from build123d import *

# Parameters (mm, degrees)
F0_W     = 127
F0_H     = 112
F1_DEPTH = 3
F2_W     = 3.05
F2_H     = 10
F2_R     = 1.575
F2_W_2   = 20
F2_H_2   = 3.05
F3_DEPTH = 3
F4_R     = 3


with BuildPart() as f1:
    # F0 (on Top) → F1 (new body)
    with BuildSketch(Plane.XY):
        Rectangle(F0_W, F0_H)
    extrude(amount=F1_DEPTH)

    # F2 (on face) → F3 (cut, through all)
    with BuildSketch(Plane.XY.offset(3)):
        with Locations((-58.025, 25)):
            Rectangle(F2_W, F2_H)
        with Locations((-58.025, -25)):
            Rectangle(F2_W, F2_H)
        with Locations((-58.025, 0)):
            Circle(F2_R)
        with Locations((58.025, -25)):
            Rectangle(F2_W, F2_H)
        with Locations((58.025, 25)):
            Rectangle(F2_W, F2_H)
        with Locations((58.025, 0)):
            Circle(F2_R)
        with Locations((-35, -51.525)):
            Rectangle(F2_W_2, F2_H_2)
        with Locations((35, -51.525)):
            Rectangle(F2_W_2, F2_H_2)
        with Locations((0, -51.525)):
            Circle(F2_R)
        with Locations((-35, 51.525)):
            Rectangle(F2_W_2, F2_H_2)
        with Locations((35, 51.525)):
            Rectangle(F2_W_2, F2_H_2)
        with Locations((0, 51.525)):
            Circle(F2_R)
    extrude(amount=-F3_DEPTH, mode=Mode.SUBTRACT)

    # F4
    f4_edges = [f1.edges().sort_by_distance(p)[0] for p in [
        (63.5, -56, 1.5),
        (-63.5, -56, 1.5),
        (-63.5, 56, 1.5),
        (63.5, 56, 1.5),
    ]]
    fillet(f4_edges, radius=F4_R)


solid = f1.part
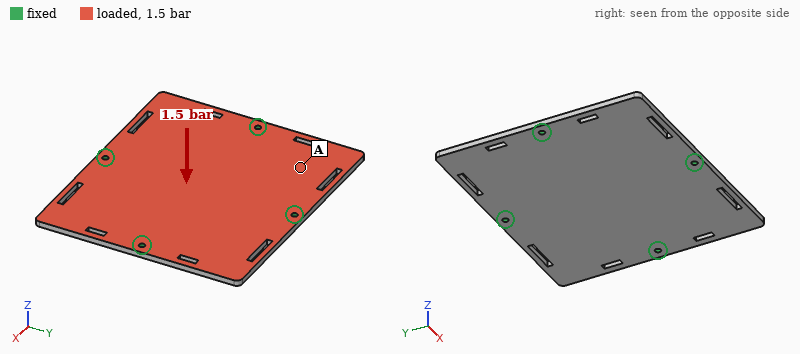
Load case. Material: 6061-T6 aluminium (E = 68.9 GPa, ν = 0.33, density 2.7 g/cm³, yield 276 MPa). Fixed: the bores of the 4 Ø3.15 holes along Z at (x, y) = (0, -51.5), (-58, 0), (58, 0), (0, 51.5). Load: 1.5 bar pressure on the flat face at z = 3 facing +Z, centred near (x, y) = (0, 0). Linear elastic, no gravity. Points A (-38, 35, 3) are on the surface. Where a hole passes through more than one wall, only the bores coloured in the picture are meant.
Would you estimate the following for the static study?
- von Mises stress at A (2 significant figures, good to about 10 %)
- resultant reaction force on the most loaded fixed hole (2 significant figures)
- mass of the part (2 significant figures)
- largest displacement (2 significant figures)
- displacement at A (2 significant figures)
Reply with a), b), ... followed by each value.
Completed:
a) 38 MPa
b) 520 N
c) 110 g
d) 0.38 mm
e) 0.19 mm
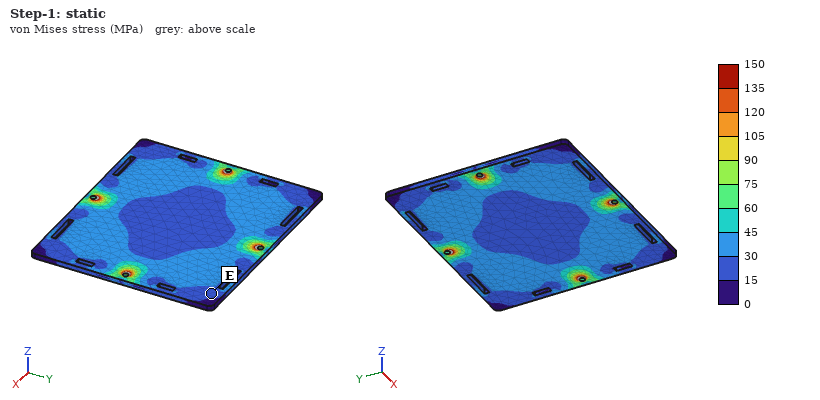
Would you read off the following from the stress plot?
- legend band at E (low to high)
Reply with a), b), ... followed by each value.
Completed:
a) 15 to 30 MPa
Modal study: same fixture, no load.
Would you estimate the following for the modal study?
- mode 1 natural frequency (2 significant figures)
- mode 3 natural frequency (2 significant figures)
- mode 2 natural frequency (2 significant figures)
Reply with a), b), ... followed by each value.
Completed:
a) 1200 Hz
b) 1400 Hz
c) 1300 Hz
